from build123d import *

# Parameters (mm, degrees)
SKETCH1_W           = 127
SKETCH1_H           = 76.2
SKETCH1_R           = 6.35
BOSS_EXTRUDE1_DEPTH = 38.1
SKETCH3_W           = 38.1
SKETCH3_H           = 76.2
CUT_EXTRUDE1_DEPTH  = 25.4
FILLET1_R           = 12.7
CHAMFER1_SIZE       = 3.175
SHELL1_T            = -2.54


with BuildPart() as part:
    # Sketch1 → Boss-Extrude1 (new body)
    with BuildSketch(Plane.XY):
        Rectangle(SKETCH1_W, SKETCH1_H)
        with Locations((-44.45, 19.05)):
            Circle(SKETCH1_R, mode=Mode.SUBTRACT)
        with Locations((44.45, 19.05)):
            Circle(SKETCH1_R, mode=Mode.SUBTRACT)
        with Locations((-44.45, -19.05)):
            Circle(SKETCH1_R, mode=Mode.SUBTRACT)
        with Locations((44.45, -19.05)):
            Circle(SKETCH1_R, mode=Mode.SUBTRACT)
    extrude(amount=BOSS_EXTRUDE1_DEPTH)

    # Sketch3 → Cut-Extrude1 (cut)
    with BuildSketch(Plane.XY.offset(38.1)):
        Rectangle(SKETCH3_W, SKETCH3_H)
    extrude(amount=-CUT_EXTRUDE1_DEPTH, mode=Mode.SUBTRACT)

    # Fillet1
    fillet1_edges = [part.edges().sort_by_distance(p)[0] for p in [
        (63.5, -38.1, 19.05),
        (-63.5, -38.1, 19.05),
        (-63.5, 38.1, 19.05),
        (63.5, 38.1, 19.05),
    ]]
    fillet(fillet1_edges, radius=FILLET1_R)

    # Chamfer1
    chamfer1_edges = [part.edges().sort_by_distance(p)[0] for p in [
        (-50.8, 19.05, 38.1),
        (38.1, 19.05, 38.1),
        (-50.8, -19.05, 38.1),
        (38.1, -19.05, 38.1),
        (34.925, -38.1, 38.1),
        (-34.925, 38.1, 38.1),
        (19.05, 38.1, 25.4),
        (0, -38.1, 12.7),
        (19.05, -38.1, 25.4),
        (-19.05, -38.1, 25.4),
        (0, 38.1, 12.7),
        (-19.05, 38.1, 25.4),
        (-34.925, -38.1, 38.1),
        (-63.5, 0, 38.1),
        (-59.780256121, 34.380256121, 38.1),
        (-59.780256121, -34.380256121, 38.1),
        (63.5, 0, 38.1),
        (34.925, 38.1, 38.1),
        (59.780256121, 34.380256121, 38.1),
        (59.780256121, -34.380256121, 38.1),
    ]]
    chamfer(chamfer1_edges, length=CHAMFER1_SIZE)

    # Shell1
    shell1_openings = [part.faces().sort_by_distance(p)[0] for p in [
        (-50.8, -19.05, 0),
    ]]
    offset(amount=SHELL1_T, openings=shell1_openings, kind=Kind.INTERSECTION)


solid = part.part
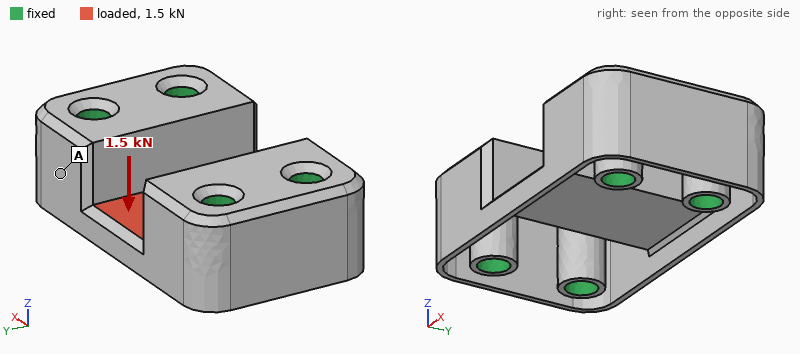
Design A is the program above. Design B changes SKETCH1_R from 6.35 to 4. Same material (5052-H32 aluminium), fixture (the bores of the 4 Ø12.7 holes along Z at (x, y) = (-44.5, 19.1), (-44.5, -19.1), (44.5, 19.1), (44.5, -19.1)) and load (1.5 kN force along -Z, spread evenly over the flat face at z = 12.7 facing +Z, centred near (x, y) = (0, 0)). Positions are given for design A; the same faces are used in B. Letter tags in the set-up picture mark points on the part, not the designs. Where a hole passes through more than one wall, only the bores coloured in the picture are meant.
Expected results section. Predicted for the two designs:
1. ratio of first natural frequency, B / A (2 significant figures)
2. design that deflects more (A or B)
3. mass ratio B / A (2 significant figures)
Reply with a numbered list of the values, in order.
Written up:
1. 0.93
2. B
3. 0.94
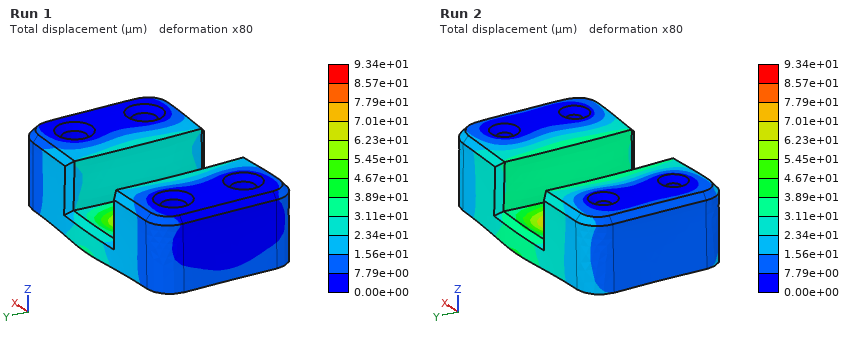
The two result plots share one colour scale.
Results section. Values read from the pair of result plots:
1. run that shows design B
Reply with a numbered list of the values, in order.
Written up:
1. Run 2
